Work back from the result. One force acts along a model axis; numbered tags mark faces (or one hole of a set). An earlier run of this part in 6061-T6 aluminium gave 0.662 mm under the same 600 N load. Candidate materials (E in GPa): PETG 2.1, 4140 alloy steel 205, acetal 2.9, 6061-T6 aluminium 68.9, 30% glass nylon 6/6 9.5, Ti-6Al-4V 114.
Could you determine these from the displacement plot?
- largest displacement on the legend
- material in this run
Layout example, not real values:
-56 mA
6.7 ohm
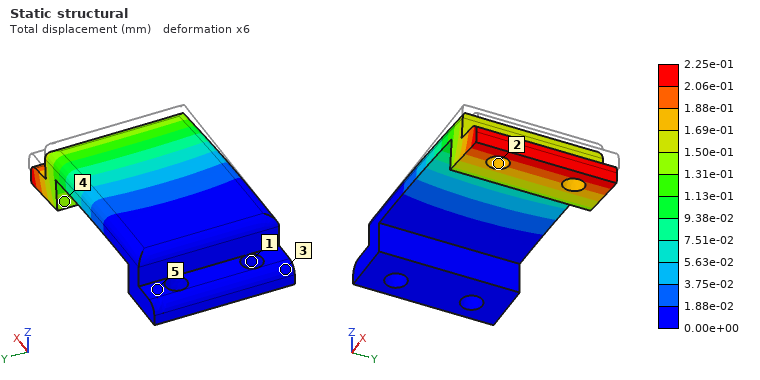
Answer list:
2.25e-01 mm
4140 alloy steel
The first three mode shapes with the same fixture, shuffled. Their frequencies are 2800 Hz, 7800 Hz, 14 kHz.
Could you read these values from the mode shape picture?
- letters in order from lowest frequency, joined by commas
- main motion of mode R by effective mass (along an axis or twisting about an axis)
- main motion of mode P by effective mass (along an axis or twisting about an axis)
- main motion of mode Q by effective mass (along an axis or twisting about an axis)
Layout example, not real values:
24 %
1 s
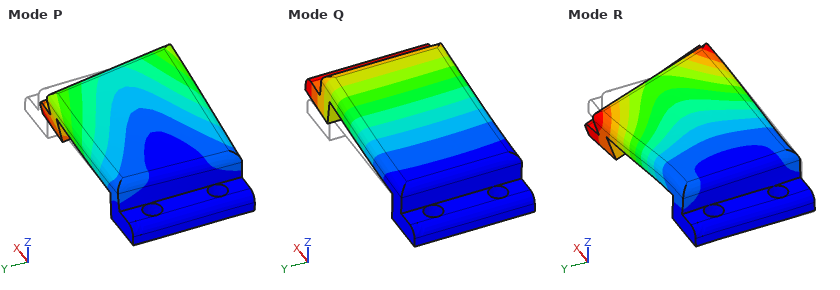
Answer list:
Q, P, R
along Y
along Y
along Z
